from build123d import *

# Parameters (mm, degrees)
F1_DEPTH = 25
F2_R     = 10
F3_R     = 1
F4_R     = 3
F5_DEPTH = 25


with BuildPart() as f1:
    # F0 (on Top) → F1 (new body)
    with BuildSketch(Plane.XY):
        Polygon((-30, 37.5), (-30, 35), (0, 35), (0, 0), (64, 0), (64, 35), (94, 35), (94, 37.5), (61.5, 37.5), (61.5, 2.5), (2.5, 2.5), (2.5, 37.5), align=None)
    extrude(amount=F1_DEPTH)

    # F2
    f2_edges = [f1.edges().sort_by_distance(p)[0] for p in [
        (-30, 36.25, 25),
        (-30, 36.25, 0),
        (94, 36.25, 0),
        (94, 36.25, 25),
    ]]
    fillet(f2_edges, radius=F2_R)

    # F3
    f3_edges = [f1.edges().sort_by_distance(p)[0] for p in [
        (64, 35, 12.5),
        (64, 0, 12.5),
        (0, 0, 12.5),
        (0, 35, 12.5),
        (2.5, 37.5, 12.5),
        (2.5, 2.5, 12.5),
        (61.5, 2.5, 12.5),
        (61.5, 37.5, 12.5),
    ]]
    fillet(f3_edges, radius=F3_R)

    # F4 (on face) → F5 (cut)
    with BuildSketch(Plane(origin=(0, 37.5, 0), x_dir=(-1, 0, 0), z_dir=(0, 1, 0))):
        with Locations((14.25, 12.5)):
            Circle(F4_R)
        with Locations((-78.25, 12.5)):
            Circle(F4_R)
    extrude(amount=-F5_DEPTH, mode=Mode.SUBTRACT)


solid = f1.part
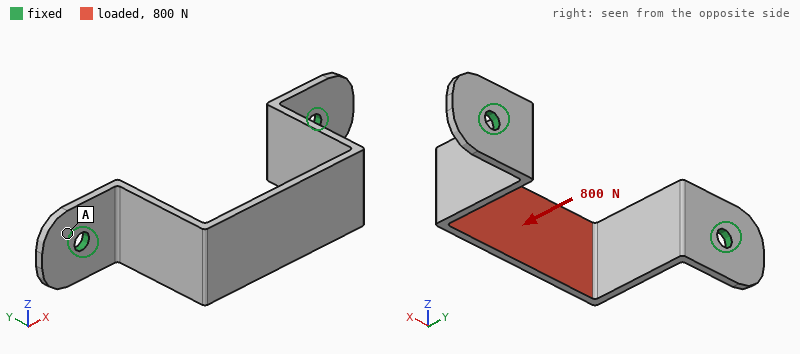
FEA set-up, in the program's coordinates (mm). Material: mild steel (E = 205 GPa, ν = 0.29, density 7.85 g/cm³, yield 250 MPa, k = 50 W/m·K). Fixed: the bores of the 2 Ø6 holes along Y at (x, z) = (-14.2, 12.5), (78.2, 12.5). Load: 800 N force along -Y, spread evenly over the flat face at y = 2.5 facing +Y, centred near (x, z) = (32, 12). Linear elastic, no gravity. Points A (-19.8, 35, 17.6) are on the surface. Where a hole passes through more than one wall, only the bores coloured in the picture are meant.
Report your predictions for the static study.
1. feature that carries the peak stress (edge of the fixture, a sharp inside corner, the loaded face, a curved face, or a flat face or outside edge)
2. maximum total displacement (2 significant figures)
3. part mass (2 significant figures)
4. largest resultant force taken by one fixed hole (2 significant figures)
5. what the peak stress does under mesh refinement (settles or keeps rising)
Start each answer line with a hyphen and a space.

- edge of the fixture
- 0.15 mm
- 92 g
- 440 N
- keeps rising
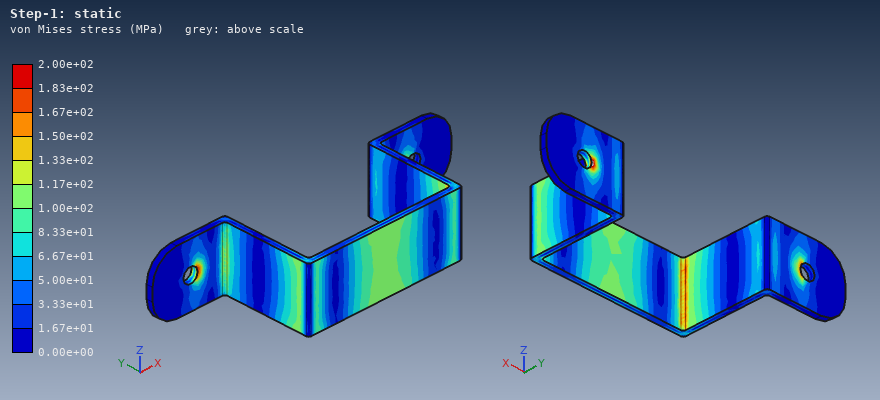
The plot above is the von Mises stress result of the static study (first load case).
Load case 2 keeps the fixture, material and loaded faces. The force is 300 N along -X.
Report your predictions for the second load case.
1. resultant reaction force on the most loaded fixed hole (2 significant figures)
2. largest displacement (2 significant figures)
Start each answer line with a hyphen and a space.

- 170 N
- 0.19 mm
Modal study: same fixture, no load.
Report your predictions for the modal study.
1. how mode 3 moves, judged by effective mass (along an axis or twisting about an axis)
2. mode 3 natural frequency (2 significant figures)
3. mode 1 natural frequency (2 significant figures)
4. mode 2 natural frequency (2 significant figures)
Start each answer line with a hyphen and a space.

- twisting about Y
- 1600 Hz
- 950 Hz
- 970 Hz
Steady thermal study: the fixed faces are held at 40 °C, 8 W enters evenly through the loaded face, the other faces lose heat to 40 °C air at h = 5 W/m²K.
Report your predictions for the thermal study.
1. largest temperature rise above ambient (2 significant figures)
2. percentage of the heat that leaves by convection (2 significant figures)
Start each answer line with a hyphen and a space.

- 72 K
- 17 %
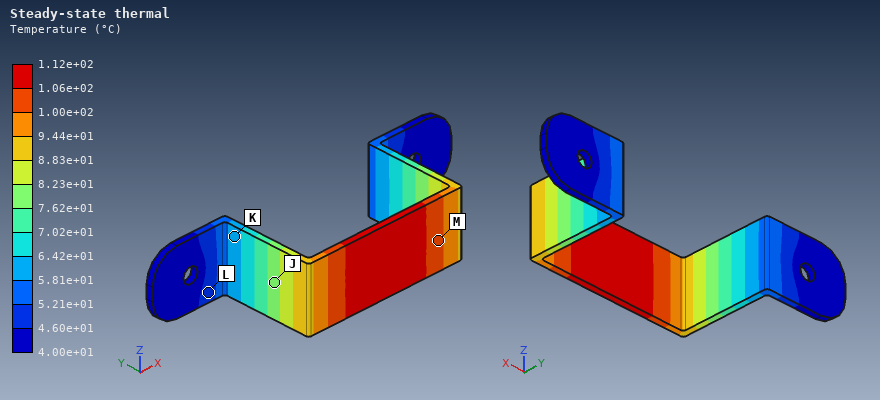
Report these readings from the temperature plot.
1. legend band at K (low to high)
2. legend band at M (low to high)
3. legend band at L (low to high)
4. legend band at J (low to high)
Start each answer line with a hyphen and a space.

- 5.81e+01 to 6.42e+01 °C
- 1.00e+02 to 1.06e+02 °C
- 4.60e+01 to 5.21e+01 °C
- 7.62e+01 to 8.23e+01 °C
